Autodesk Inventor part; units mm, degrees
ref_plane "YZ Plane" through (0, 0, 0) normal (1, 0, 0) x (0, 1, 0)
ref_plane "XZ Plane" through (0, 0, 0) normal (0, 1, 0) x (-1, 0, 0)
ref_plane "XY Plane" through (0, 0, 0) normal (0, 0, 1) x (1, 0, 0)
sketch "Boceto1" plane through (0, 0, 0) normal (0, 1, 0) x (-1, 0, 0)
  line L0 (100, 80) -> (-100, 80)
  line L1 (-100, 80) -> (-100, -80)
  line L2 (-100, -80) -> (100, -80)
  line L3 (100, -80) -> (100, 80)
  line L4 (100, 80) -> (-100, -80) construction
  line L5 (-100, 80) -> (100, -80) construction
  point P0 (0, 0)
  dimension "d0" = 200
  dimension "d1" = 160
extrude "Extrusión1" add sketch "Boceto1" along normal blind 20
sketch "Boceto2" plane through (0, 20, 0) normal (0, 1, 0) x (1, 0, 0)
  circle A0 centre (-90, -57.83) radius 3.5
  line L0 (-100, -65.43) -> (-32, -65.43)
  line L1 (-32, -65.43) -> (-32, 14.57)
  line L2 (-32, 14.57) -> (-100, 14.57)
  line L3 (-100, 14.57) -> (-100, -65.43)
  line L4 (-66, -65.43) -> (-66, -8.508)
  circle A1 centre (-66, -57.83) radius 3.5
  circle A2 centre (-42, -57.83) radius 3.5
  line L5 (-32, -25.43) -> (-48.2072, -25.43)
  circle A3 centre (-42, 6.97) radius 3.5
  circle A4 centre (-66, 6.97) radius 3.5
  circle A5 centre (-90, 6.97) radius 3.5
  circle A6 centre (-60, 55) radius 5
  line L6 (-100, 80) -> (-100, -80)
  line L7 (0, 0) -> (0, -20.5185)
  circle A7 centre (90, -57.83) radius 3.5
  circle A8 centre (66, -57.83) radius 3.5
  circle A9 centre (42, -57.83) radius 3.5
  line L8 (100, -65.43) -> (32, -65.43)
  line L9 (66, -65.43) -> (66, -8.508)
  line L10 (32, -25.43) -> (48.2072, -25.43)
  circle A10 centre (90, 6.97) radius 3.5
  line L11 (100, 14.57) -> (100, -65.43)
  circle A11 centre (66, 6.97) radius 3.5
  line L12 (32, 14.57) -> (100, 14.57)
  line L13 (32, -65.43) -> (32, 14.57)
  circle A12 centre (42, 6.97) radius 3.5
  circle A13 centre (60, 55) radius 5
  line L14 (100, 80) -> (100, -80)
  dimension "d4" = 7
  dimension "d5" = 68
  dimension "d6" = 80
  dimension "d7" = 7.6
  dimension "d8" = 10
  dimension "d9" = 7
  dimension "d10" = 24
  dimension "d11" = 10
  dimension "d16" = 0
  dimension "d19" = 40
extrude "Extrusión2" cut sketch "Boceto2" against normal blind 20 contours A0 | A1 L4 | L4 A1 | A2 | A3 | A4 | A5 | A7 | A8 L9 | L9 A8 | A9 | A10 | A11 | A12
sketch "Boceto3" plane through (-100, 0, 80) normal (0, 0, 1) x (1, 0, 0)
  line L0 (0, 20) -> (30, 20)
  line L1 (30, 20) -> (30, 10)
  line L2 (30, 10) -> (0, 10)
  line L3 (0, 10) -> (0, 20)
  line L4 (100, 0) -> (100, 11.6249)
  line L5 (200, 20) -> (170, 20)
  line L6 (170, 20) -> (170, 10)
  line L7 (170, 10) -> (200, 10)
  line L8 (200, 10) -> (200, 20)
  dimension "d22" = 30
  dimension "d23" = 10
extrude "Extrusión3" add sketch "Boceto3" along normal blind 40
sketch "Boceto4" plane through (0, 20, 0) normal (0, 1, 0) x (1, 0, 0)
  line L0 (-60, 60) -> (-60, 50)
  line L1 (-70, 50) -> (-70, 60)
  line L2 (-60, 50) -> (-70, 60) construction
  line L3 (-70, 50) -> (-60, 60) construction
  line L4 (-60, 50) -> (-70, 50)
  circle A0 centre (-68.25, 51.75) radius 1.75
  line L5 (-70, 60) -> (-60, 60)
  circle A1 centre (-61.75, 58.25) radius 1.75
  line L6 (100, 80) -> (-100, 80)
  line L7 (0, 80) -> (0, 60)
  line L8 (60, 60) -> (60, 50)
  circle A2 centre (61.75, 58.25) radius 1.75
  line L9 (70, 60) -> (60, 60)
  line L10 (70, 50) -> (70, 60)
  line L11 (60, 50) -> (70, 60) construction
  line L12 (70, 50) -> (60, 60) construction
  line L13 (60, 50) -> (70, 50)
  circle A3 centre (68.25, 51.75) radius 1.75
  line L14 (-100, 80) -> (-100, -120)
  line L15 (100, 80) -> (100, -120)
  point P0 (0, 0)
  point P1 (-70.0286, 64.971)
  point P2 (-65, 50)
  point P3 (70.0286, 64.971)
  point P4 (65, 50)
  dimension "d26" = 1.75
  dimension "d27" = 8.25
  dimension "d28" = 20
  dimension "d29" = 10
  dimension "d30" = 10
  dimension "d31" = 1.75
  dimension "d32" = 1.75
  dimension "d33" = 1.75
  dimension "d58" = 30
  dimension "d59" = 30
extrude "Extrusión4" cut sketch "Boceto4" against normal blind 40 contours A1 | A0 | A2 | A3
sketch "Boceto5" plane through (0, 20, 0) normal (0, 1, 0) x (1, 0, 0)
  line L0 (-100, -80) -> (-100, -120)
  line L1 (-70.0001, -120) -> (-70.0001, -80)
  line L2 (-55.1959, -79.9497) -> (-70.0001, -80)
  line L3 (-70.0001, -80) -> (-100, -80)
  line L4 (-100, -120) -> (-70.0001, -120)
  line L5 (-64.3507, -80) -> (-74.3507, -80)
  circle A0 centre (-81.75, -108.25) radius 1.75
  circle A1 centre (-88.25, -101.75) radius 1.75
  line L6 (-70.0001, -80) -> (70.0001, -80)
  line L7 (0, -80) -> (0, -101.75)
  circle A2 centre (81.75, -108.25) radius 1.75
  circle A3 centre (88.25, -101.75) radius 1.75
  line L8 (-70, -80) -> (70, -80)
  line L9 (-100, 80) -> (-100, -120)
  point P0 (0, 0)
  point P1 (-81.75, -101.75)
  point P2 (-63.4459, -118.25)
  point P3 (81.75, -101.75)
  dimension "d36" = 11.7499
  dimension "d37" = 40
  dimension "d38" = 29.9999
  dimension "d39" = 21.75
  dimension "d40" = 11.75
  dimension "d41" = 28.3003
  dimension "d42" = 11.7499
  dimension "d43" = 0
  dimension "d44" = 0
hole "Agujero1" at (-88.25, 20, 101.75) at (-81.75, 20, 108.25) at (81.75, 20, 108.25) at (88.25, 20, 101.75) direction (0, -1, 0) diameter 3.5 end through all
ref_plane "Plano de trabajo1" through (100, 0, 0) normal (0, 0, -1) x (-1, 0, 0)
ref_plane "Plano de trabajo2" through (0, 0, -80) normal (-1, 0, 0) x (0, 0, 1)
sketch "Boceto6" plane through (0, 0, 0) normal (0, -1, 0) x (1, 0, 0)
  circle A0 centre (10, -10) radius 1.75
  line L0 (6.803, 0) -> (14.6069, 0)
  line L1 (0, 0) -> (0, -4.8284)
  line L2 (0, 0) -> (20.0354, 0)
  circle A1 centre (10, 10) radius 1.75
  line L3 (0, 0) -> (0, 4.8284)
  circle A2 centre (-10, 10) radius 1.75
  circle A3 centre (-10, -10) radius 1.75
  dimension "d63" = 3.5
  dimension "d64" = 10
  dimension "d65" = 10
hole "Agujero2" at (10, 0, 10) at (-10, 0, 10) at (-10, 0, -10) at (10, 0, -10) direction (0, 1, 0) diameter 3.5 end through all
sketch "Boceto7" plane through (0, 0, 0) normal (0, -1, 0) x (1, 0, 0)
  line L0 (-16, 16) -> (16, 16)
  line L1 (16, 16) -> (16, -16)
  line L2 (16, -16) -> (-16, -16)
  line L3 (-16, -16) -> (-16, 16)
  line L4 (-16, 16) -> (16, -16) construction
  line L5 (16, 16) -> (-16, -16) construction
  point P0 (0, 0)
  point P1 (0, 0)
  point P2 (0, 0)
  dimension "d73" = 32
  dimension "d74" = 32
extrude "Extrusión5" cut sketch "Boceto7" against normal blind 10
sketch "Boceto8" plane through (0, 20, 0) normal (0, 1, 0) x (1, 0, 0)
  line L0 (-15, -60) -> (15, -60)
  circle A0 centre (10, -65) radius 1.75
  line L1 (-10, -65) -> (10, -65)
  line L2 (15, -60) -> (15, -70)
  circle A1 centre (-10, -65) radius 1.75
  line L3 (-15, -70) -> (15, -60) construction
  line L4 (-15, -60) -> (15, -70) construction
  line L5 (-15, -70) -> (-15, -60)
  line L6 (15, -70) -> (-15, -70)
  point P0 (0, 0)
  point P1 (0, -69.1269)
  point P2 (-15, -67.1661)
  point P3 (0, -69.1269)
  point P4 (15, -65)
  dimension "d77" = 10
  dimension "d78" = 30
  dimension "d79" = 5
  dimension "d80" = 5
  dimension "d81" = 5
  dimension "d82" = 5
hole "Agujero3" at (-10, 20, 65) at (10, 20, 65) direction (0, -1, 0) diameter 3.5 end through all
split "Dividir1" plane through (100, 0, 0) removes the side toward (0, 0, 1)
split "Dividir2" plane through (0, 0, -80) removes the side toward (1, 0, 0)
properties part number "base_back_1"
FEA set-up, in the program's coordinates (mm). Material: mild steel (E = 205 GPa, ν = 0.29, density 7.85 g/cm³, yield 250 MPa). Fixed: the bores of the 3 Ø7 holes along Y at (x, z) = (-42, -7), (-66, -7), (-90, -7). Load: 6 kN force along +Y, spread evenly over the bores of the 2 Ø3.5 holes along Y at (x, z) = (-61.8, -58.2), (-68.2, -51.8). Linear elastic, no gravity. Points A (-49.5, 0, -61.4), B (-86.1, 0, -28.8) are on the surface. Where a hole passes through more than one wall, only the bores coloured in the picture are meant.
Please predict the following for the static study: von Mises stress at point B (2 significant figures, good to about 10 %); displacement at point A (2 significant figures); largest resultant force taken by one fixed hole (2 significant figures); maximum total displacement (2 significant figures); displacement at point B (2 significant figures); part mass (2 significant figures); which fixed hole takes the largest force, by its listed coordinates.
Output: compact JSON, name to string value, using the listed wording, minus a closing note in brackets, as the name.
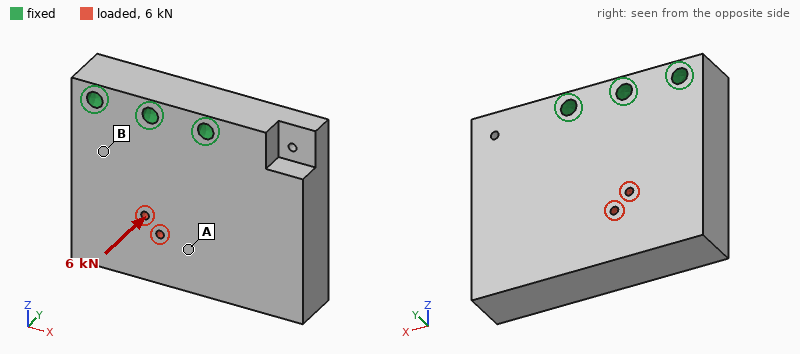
{"von Mises stress at point B": "30 MPa", "displacement at point A": "29 µm", "largest resultant force taken by one fixed hole": "2.8 kN", "maximum total displacement": "42 µm", "displacement at point B": "8.7 µm", "part mass": "1.2 kg", "which fixed hole takes the largest force, by its listed coordinates": "(-66, -7)"}
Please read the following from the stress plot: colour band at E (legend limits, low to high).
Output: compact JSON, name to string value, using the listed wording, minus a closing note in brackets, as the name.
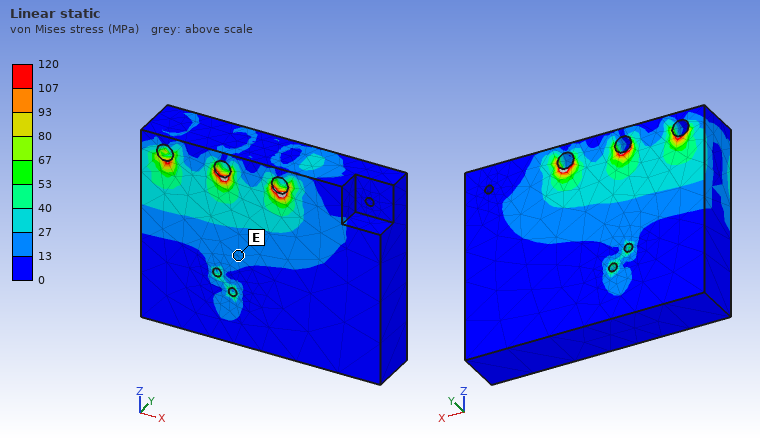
{"colour band at E": "13 to 27 MPa"}
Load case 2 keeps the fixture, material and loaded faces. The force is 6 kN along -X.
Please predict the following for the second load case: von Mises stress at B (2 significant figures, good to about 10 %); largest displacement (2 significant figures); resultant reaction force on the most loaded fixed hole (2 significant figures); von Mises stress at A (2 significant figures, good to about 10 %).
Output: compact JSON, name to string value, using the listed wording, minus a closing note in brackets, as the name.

{"von Mises stress at B": "10 MPa", "largest displacement": "8.2 µm", "resultant reaction force on the most loaded fixed hole": "5.7 kN", "von Mises stress at A": "3.7 MPa"}
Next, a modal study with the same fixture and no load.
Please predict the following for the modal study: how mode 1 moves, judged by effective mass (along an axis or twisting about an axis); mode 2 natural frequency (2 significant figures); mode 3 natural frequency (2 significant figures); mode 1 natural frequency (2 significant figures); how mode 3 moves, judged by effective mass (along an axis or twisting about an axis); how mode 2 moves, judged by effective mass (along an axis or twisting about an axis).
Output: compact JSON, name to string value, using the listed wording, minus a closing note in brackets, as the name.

{"how mode 1 moves, judged by effective mass": "along Y", "mode 2 natural frequency": "4300 Hz", "mode 3 natural frequency": "5200 Hz", "mode 1 natural frequency": "2500 Hz", "how mode 3 moves, judged by effective mass": "along X", "how mode 2 moves, judged by effective mass": "twisting about Z"}
